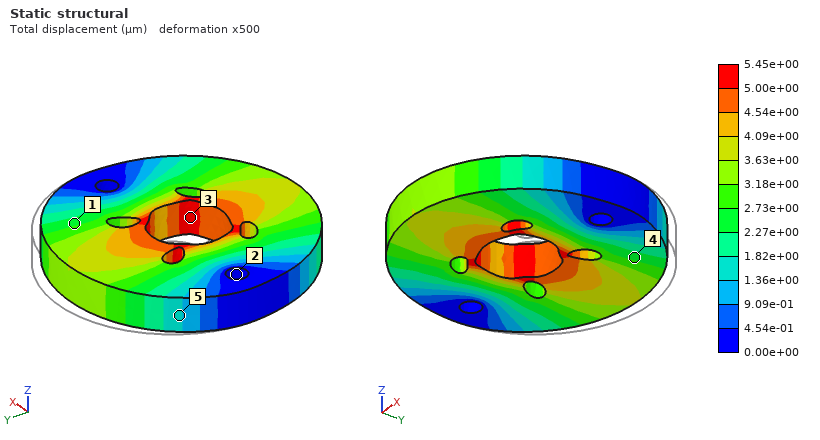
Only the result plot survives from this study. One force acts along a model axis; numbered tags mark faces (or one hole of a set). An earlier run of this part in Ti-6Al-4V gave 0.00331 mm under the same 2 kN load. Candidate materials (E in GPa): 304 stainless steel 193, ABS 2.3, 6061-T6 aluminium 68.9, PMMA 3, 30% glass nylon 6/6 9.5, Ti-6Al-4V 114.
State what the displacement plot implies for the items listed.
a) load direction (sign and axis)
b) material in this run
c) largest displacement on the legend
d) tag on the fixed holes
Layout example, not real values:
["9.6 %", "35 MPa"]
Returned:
["-Y", "6061-T6 aluminium", "5.45e+00 µm", "2"]
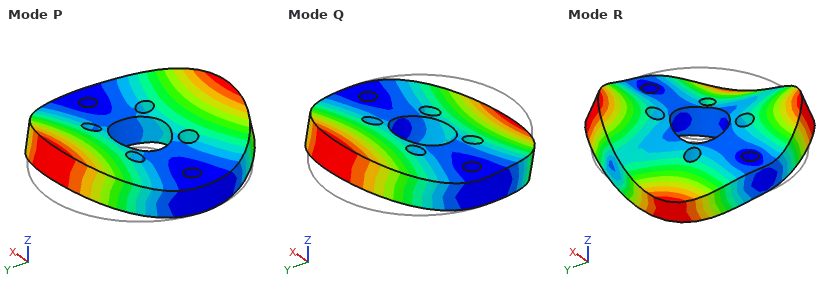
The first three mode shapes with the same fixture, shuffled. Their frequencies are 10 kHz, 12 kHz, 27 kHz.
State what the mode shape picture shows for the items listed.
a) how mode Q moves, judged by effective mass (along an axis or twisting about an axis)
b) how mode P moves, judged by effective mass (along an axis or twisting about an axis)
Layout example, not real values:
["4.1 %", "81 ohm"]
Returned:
["twisting about X", "along Z"]
